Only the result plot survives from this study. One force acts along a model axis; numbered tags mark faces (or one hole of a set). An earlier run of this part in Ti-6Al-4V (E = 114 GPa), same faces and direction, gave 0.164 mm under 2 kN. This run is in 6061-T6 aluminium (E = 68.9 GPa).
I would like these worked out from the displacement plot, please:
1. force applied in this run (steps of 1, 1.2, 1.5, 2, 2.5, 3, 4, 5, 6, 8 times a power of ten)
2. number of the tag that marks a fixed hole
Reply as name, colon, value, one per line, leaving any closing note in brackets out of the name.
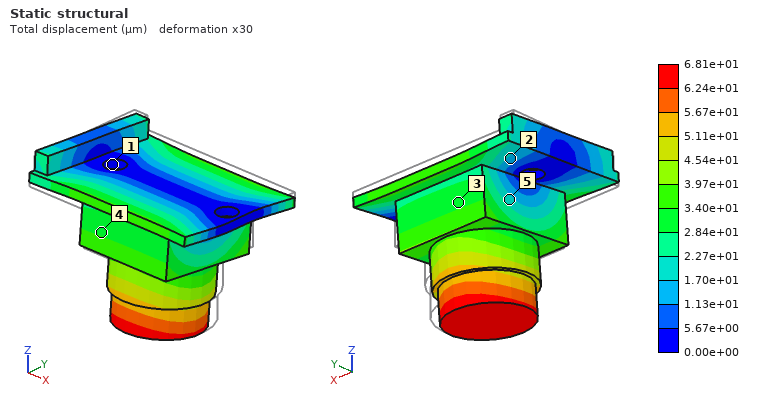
force applied in this run: 500 N
number of the tag that marks a fixed hole: 1
